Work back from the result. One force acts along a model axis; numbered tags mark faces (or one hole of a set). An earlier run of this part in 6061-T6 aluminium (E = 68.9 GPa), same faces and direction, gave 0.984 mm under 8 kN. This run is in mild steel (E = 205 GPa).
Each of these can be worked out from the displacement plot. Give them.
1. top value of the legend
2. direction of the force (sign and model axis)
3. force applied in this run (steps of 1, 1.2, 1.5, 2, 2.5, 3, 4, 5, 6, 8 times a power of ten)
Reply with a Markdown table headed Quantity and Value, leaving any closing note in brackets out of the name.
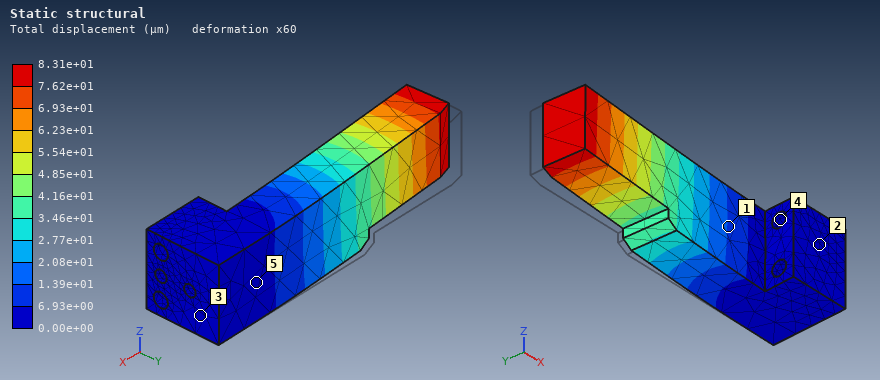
| Quantity | Value |
|---|---|
| top value of the legend | 8.31e+01 µm |
| direction of the force | -Y |
| force applied in this run | 2 kN |
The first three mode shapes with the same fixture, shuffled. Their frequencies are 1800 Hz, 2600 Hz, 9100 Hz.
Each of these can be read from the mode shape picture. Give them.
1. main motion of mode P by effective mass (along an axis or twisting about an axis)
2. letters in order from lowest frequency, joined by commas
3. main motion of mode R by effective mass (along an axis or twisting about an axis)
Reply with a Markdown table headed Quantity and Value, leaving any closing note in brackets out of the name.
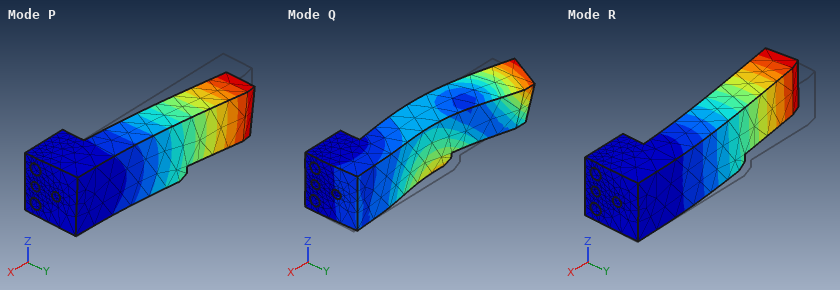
| Quantity | Value |
|---|---|
| main motion of mode P by effective mass | along Z |
| letters in order from lowest frequency, joined by commas | R, P, Q |
| main motion of mode R by effective mass | along Y |
